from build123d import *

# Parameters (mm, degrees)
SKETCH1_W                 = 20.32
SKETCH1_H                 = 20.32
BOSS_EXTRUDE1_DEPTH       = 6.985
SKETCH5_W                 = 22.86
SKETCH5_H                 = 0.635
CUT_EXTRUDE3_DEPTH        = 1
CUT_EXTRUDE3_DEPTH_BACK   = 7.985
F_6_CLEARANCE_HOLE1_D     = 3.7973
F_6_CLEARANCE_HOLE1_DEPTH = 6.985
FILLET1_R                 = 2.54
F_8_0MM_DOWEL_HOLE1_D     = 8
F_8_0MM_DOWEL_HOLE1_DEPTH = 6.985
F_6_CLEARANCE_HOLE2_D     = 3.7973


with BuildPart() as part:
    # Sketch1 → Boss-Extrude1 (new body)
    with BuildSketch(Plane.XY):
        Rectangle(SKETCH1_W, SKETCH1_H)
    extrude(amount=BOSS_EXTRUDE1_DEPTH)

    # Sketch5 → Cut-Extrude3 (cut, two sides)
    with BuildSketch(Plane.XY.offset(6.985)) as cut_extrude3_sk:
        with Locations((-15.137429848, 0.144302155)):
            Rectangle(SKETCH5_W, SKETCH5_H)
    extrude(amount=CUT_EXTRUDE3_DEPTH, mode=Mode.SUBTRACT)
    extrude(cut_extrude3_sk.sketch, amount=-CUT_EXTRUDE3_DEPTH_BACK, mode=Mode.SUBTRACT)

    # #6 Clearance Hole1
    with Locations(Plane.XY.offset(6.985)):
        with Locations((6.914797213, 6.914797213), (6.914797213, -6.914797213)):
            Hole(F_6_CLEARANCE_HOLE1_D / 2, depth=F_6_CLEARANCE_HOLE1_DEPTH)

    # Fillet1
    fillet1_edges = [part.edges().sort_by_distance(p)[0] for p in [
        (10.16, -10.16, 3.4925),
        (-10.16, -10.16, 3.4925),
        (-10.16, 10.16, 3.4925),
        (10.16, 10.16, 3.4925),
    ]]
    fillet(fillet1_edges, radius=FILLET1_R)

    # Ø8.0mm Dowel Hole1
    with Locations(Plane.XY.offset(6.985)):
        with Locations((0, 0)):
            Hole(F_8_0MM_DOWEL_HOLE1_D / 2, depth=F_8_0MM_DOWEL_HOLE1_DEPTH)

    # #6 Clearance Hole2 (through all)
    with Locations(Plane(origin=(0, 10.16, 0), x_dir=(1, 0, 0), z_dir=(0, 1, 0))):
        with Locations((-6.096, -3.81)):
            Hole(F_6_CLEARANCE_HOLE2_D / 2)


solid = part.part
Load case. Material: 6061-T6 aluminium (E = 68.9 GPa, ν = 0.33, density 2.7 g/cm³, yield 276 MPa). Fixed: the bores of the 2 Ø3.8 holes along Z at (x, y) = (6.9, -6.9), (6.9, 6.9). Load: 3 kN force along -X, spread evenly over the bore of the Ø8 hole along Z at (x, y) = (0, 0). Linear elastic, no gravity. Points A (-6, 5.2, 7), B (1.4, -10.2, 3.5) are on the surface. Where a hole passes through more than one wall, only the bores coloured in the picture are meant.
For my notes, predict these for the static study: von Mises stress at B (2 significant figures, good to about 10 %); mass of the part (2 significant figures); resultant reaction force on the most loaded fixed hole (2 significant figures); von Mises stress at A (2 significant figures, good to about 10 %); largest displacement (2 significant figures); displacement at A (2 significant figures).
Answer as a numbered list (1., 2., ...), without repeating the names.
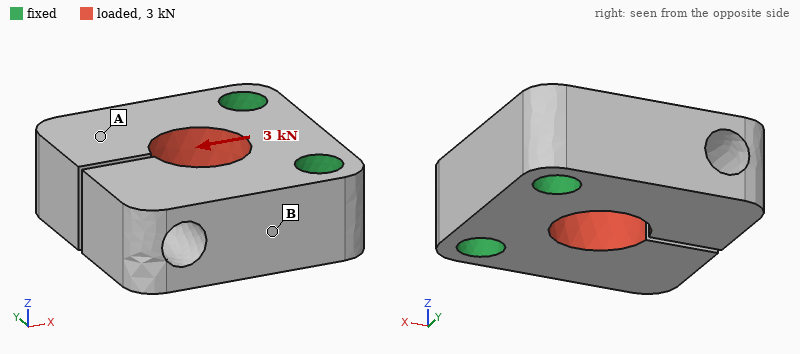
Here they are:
1. 54 MPa
2. 5.6 g
3. 1.5 kN
4. 21 MPa
5. 47 µm
6. 25 µm
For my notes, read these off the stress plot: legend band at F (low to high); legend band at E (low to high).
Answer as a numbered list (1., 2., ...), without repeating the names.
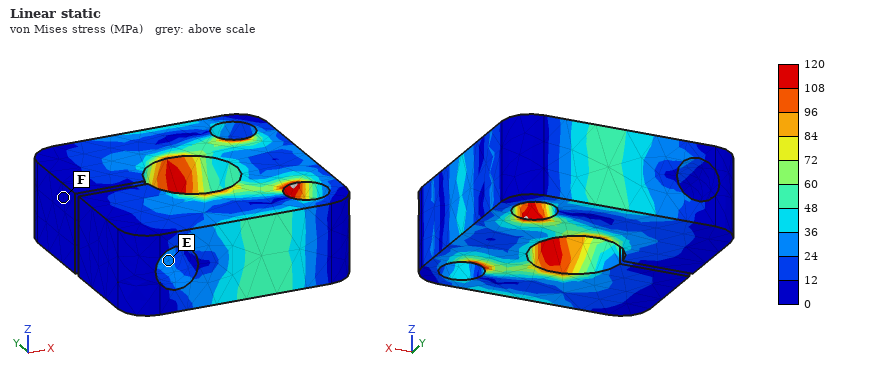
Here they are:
1. 0 to 12 MPa
2. 24 to 36 MPa
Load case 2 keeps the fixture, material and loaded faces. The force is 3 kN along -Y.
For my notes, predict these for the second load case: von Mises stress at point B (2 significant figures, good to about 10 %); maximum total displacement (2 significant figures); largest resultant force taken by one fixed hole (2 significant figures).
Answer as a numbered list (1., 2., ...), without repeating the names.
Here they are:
1. 54 MPa
2. 41 µm
3. 1.7 kN
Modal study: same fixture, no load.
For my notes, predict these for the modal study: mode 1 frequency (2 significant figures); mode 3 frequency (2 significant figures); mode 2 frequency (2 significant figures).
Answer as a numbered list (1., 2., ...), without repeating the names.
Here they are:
1. 17 kHz
2. 18 kHz
3. 18 kHz
